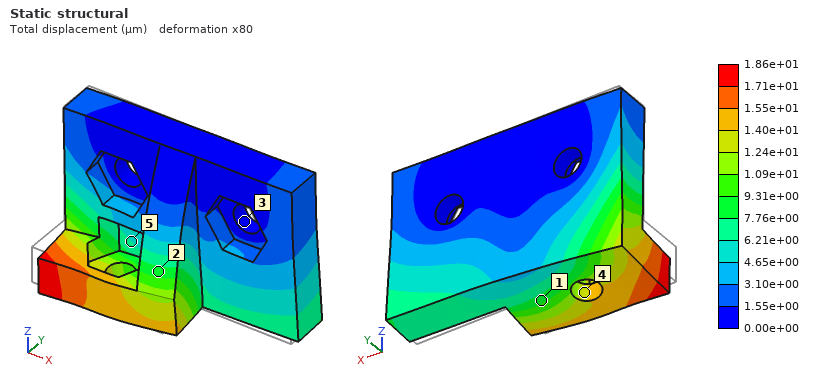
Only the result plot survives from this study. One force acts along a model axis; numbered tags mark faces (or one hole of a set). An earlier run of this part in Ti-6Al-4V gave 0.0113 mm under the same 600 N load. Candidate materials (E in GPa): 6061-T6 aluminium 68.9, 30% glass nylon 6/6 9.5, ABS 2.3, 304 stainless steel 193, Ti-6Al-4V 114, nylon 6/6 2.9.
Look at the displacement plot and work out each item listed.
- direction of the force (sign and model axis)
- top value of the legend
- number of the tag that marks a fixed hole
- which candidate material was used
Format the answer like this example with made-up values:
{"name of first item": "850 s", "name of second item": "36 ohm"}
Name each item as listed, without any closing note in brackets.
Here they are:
{"direction of the force": "+X", "top value of the legend": "1.86e+01 µm", "number of the tag that marks a fixed hole": "3", "which candidate material was used": "6061-T6 aluminium"}
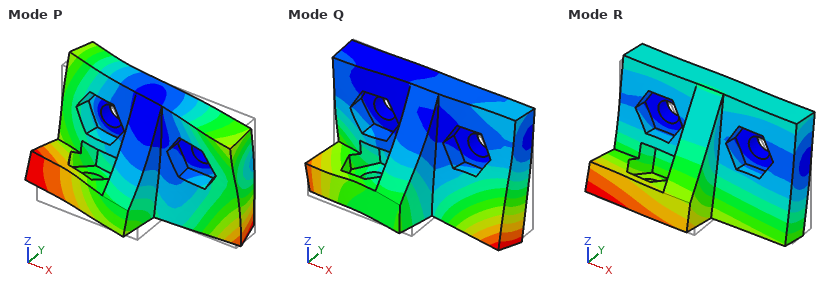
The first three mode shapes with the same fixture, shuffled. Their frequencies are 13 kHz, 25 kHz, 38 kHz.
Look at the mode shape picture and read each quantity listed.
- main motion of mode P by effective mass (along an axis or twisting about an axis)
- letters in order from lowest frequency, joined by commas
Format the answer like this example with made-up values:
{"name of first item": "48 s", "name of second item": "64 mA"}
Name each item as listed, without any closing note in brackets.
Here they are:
{"main motion of mode P by effective mass": "along X", "letters in order from lowest frequency, joined by commas": "R, Q, P"}
